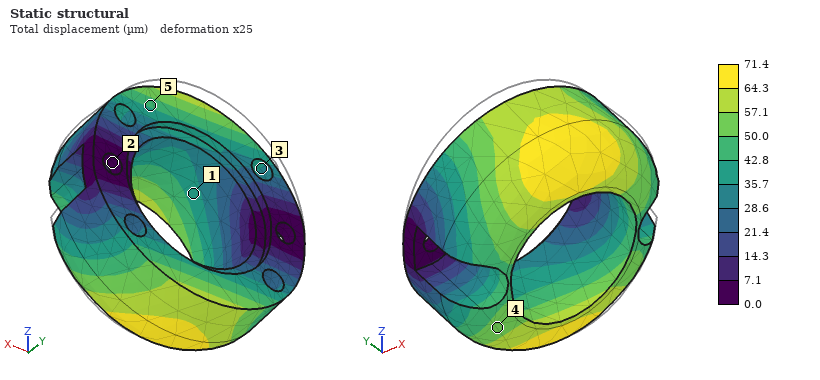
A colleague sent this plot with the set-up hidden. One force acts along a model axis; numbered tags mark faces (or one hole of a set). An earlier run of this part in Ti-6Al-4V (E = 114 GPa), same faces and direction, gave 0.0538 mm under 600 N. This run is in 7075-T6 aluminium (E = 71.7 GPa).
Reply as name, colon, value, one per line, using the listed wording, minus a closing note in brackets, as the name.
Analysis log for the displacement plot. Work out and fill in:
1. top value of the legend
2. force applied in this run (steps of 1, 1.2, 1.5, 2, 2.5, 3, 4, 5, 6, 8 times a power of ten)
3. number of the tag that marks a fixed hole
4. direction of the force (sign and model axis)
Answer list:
top value of the legend: 71.4 µm
force applied in this run: 500 N
number of the tag that marks a fixed hole: 2
direction of the force: -Z
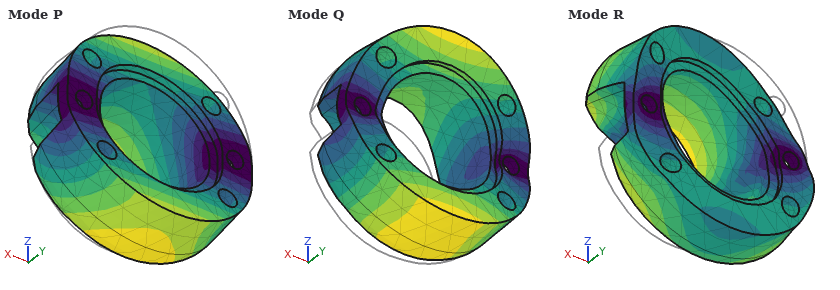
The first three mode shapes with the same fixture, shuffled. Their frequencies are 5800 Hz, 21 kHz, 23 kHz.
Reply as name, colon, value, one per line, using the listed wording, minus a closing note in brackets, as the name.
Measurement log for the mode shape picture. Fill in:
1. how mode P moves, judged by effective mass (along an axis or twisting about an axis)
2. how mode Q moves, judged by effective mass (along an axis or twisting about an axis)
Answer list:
how mode P moves, judged by effective mass: along Z
how mode Q moves, judged by effective mass: along Y
